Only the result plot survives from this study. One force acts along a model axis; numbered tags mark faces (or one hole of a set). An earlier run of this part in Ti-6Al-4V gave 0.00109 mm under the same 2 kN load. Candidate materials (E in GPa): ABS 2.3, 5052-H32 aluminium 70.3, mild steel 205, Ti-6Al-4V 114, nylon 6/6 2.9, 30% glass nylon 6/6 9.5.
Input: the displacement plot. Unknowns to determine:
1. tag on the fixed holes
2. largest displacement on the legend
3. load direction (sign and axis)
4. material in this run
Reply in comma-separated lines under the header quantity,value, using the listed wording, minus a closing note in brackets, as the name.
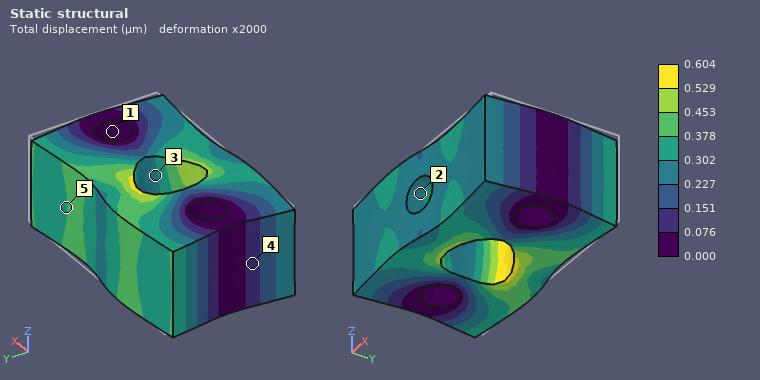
quantity,value
tag on the fixed holes,1
largest displacement on the legend,0.604 µm
load direction,-X
material in this run,mild steel
